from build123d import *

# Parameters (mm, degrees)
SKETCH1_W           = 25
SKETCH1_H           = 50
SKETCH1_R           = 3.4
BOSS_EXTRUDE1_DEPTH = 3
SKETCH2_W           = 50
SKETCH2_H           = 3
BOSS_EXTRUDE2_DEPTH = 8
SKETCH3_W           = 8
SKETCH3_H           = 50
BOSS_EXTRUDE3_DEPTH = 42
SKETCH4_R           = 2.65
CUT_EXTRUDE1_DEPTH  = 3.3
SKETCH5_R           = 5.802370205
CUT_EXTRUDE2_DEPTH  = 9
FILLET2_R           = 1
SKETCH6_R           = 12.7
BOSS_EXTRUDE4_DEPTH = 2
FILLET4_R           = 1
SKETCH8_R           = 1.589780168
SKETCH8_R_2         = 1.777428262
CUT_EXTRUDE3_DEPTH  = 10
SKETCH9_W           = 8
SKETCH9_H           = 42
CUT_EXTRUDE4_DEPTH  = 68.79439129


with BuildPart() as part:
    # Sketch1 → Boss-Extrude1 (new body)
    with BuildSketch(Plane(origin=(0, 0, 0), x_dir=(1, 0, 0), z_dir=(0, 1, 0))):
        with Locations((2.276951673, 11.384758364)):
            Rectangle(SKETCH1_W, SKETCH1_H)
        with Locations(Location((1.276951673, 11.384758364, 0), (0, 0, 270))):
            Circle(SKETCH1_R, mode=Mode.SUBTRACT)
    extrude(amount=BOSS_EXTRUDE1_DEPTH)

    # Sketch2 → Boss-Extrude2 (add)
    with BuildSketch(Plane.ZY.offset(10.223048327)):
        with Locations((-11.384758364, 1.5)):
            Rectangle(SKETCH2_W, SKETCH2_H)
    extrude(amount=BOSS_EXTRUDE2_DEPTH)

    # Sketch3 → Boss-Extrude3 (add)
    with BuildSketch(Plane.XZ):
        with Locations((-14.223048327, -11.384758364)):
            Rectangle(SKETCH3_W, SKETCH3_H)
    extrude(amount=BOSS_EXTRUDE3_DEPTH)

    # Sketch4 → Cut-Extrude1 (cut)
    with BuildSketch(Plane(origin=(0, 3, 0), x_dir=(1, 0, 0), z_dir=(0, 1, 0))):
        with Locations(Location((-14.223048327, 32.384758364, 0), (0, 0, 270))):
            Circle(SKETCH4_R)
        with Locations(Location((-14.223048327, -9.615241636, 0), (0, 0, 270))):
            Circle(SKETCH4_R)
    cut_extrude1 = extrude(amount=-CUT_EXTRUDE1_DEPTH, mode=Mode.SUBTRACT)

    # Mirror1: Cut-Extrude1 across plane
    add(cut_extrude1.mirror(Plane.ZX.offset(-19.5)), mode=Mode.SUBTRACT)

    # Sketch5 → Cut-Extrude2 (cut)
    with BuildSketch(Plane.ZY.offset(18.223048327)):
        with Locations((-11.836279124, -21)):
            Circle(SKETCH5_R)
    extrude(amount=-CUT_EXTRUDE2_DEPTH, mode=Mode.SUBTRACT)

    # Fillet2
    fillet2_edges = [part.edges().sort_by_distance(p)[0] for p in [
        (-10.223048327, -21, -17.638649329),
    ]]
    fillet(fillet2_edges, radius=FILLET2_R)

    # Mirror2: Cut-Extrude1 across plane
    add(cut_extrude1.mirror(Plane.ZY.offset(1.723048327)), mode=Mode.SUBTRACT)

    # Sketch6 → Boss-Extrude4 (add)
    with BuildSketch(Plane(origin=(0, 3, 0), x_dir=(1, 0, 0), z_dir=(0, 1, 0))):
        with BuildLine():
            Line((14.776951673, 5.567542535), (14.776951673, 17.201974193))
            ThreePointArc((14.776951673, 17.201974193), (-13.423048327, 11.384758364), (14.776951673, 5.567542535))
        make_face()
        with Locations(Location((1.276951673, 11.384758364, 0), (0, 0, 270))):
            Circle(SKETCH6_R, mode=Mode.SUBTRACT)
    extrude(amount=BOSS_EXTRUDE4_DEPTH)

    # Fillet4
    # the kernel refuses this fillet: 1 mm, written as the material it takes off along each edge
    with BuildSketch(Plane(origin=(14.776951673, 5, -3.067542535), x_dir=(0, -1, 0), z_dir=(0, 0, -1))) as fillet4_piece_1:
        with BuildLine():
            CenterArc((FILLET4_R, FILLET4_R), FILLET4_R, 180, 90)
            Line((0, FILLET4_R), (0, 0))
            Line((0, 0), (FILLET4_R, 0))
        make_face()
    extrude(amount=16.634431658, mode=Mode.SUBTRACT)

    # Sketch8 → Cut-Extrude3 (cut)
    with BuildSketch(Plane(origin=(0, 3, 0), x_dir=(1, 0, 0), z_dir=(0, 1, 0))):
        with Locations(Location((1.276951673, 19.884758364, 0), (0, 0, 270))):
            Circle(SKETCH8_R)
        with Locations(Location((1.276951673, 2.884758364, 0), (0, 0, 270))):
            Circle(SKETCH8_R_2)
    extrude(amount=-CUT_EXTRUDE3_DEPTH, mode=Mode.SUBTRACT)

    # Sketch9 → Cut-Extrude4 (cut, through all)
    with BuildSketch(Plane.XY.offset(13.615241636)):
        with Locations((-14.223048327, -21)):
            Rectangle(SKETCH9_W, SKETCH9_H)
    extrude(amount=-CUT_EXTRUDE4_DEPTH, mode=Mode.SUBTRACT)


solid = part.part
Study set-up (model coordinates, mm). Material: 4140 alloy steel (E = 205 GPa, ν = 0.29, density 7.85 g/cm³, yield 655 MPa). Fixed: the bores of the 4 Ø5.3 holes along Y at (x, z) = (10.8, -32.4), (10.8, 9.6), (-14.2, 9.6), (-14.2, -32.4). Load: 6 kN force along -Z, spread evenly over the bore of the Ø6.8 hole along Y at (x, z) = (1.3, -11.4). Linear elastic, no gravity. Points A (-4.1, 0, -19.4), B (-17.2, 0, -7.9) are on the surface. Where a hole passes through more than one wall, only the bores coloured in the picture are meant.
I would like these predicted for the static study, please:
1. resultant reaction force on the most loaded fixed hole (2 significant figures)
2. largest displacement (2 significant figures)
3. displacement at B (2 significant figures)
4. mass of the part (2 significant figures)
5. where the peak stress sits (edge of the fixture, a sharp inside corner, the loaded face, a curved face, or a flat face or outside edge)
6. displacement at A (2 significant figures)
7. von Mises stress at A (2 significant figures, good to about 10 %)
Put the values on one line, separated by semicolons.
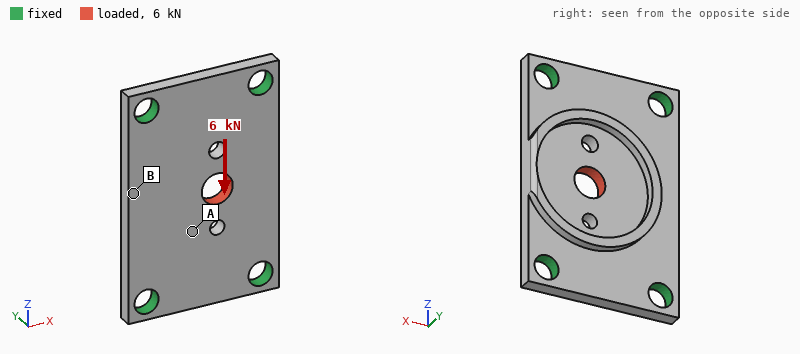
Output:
1.8 kN; 6.8 µm; 1.2 µm; 38 g; a curved face; 3.4 µm; 47 MPa
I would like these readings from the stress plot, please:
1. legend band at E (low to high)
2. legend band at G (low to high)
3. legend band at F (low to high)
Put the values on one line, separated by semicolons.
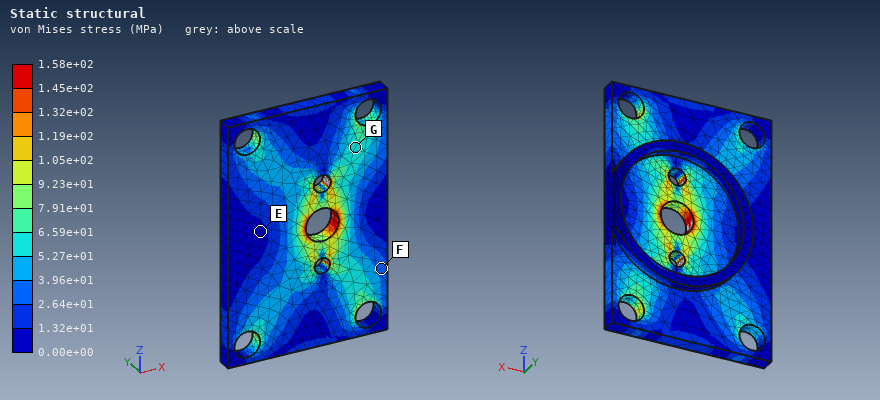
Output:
0.00e+00 to 1.32e+01 MPa; 5.27e+01 to 6.59e+01 MPa; 2.64e+01 to 3.96e+01 MPa
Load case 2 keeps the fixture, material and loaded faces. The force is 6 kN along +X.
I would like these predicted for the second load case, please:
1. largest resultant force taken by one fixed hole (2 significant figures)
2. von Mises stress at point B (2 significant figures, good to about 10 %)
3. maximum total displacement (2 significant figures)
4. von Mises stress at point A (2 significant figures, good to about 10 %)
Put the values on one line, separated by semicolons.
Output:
1.9 kN; 37 MPa; 12 µm; 80 MPa
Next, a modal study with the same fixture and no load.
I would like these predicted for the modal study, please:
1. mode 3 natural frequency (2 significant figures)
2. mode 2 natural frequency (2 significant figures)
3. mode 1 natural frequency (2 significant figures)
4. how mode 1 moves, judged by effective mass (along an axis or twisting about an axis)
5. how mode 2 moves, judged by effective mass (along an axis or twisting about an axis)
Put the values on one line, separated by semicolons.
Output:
22 kHz; 13 kHz; 9600 Hz; along Y; twisting about Z
